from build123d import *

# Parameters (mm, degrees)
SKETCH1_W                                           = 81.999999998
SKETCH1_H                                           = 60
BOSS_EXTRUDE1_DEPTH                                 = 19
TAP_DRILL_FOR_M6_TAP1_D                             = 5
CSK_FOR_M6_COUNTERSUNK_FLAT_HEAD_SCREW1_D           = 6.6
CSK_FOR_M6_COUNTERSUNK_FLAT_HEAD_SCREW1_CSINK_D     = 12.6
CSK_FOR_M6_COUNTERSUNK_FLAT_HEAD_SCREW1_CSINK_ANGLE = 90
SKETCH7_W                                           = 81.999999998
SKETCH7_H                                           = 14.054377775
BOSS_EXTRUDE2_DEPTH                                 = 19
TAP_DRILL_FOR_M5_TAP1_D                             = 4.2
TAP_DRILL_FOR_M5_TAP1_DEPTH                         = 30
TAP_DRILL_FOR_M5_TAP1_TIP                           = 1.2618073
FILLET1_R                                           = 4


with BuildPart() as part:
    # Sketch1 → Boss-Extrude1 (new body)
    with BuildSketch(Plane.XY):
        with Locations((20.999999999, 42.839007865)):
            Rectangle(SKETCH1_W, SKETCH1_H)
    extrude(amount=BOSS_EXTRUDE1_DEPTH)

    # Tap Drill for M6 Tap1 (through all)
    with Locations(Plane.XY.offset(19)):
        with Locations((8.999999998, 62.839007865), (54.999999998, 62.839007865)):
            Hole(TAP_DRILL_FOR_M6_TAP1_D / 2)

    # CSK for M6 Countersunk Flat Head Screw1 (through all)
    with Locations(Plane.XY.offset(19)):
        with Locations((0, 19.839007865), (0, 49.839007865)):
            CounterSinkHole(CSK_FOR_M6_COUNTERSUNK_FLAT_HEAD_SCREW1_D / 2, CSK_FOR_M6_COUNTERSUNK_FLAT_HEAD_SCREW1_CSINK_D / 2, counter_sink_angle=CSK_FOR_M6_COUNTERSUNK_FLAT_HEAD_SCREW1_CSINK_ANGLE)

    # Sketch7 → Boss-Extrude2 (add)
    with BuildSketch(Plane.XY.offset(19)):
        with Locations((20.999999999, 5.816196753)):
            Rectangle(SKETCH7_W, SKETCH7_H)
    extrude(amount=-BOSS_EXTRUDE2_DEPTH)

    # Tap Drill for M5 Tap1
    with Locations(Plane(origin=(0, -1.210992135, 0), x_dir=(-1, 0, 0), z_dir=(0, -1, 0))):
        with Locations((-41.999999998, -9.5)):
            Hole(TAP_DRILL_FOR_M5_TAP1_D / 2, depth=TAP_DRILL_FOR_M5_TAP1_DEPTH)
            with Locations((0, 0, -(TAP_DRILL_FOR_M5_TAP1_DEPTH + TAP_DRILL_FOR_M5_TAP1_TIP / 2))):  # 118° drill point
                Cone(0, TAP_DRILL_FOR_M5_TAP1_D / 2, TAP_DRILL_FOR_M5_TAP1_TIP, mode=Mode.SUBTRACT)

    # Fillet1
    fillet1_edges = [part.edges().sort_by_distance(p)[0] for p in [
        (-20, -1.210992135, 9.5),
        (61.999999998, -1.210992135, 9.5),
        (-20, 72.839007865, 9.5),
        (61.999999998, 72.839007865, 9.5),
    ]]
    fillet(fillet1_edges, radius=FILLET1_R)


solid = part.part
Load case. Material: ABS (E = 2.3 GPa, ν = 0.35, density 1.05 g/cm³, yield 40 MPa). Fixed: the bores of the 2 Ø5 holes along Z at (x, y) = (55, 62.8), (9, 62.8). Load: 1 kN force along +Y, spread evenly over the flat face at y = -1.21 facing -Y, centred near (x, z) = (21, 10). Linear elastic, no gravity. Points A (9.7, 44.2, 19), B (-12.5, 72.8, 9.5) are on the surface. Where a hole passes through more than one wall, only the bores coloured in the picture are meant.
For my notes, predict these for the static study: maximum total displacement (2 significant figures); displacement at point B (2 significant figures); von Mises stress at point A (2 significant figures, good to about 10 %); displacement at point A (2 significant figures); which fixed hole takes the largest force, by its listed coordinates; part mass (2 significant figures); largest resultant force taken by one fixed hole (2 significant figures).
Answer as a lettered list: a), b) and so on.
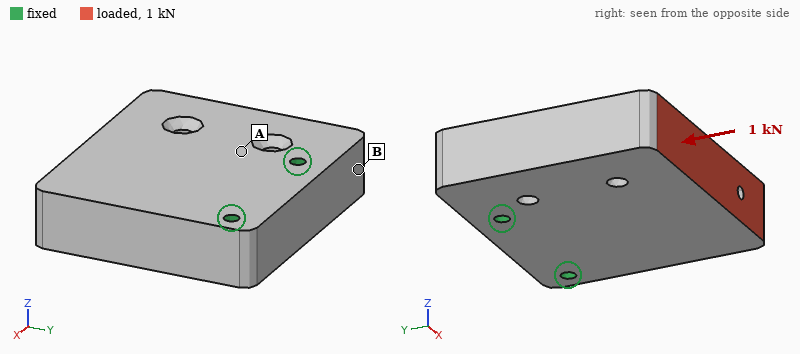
a) 42 µm
b) 24 µm
c) 1.3 MPa
d) 15 µm
e) (9, 62.8)
f) 120 g
g) 730 N
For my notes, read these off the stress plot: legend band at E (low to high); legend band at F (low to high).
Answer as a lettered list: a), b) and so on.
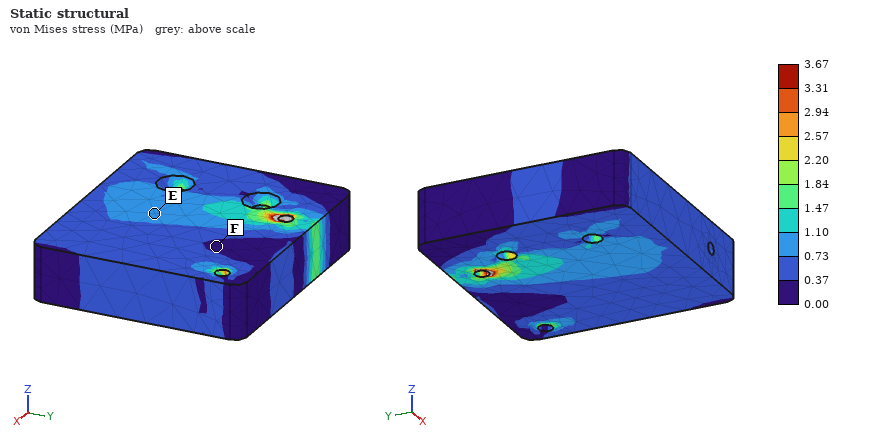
a) 0.73 to 1.10 MPa
b) 0.00 to 0.37 MPa
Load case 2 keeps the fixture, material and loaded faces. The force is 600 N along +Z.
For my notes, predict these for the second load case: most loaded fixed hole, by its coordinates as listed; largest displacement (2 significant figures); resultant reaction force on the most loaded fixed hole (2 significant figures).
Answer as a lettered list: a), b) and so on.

a) (9, 62.8)
b) 0.84 mm
c) 430 N
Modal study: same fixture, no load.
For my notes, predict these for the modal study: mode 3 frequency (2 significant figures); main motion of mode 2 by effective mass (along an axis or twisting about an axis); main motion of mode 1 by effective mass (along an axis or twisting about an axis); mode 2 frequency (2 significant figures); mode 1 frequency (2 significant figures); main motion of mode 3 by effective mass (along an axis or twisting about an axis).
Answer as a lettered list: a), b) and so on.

a) 1900 Hz
b) twisting about Y
c) along Z
d) 1600 Hz
e) 810 Hz
f) along X
